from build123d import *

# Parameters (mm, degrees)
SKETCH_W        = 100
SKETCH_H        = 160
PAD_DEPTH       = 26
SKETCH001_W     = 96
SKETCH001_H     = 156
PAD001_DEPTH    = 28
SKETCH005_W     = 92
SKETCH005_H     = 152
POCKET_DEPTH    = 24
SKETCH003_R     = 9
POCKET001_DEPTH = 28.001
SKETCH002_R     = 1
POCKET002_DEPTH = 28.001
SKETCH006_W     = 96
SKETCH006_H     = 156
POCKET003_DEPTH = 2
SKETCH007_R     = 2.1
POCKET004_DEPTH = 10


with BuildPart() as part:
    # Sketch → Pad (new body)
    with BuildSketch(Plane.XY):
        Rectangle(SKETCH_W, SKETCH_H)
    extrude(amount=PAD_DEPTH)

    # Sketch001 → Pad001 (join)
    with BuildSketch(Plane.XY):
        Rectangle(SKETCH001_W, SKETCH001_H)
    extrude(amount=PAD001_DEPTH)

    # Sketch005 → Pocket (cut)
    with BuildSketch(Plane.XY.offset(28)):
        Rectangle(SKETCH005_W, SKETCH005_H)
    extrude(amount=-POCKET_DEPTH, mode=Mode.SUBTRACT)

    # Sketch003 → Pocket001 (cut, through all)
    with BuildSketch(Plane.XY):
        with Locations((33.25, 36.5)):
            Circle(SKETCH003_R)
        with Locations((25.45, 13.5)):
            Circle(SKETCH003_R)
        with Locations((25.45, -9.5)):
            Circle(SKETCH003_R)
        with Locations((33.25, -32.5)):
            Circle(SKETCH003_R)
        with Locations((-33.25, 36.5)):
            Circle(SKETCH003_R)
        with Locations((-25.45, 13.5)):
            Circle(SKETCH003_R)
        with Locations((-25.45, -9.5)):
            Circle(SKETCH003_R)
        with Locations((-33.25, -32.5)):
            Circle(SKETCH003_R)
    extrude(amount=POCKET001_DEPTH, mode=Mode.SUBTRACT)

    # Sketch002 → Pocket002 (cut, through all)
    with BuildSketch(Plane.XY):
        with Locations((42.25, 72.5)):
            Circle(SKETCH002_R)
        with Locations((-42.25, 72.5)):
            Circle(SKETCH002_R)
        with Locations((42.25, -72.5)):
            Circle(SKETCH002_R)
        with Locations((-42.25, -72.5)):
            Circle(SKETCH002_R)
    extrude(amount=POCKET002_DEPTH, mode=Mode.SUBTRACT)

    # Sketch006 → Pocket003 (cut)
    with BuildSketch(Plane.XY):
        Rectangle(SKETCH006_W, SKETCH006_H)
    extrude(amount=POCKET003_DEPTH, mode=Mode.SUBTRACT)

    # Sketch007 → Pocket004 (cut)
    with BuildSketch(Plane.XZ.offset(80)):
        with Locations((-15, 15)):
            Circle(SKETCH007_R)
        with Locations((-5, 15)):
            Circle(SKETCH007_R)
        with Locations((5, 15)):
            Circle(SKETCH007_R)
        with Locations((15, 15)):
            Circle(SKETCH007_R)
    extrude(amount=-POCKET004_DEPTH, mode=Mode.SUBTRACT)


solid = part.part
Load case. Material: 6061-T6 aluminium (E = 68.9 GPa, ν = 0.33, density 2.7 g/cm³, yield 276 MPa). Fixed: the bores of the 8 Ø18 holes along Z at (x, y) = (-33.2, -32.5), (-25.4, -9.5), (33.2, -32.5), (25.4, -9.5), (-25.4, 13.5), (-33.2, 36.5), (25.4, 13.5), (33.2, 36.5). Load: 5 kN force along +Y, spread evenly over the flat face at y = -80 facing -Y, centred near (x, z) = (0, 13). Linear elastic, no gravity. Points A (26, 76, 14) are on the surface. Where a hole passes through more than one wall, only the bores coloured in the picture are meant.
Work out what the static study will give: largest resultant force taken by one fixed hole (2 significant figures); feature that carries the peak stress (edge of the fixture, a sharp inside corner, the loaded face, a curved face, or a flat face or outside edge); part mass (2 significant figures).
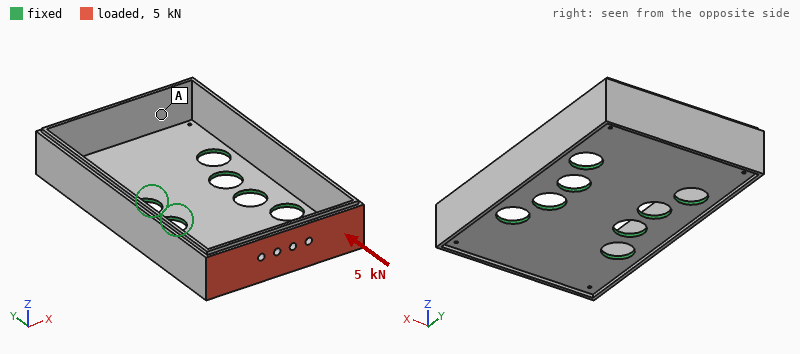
1.5 kN
a flat face or outside edge
210 g
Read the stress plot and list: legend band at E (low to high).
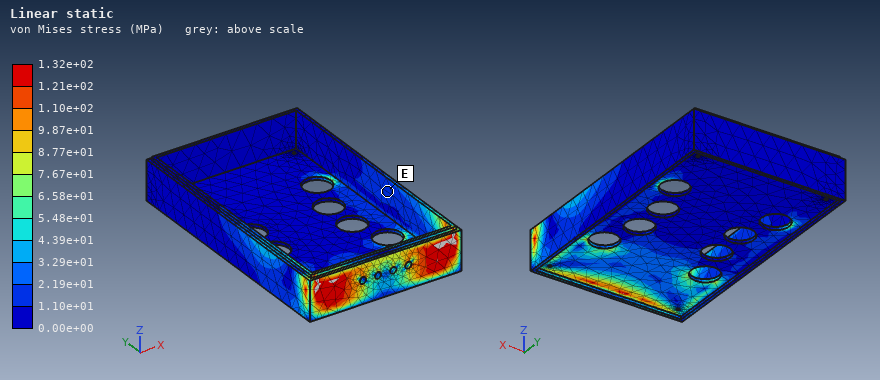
1.10e+01 to 2.19e+01 MPa
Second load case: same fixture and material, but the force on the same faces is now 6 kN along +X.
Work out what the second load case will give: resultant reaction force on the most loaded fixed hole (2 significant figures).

4.8 kN
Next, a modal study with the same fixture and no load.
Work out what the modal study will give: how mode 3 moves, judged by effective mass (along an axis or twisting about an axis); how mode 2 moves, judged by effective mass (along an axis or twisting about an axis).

along Z
along X
